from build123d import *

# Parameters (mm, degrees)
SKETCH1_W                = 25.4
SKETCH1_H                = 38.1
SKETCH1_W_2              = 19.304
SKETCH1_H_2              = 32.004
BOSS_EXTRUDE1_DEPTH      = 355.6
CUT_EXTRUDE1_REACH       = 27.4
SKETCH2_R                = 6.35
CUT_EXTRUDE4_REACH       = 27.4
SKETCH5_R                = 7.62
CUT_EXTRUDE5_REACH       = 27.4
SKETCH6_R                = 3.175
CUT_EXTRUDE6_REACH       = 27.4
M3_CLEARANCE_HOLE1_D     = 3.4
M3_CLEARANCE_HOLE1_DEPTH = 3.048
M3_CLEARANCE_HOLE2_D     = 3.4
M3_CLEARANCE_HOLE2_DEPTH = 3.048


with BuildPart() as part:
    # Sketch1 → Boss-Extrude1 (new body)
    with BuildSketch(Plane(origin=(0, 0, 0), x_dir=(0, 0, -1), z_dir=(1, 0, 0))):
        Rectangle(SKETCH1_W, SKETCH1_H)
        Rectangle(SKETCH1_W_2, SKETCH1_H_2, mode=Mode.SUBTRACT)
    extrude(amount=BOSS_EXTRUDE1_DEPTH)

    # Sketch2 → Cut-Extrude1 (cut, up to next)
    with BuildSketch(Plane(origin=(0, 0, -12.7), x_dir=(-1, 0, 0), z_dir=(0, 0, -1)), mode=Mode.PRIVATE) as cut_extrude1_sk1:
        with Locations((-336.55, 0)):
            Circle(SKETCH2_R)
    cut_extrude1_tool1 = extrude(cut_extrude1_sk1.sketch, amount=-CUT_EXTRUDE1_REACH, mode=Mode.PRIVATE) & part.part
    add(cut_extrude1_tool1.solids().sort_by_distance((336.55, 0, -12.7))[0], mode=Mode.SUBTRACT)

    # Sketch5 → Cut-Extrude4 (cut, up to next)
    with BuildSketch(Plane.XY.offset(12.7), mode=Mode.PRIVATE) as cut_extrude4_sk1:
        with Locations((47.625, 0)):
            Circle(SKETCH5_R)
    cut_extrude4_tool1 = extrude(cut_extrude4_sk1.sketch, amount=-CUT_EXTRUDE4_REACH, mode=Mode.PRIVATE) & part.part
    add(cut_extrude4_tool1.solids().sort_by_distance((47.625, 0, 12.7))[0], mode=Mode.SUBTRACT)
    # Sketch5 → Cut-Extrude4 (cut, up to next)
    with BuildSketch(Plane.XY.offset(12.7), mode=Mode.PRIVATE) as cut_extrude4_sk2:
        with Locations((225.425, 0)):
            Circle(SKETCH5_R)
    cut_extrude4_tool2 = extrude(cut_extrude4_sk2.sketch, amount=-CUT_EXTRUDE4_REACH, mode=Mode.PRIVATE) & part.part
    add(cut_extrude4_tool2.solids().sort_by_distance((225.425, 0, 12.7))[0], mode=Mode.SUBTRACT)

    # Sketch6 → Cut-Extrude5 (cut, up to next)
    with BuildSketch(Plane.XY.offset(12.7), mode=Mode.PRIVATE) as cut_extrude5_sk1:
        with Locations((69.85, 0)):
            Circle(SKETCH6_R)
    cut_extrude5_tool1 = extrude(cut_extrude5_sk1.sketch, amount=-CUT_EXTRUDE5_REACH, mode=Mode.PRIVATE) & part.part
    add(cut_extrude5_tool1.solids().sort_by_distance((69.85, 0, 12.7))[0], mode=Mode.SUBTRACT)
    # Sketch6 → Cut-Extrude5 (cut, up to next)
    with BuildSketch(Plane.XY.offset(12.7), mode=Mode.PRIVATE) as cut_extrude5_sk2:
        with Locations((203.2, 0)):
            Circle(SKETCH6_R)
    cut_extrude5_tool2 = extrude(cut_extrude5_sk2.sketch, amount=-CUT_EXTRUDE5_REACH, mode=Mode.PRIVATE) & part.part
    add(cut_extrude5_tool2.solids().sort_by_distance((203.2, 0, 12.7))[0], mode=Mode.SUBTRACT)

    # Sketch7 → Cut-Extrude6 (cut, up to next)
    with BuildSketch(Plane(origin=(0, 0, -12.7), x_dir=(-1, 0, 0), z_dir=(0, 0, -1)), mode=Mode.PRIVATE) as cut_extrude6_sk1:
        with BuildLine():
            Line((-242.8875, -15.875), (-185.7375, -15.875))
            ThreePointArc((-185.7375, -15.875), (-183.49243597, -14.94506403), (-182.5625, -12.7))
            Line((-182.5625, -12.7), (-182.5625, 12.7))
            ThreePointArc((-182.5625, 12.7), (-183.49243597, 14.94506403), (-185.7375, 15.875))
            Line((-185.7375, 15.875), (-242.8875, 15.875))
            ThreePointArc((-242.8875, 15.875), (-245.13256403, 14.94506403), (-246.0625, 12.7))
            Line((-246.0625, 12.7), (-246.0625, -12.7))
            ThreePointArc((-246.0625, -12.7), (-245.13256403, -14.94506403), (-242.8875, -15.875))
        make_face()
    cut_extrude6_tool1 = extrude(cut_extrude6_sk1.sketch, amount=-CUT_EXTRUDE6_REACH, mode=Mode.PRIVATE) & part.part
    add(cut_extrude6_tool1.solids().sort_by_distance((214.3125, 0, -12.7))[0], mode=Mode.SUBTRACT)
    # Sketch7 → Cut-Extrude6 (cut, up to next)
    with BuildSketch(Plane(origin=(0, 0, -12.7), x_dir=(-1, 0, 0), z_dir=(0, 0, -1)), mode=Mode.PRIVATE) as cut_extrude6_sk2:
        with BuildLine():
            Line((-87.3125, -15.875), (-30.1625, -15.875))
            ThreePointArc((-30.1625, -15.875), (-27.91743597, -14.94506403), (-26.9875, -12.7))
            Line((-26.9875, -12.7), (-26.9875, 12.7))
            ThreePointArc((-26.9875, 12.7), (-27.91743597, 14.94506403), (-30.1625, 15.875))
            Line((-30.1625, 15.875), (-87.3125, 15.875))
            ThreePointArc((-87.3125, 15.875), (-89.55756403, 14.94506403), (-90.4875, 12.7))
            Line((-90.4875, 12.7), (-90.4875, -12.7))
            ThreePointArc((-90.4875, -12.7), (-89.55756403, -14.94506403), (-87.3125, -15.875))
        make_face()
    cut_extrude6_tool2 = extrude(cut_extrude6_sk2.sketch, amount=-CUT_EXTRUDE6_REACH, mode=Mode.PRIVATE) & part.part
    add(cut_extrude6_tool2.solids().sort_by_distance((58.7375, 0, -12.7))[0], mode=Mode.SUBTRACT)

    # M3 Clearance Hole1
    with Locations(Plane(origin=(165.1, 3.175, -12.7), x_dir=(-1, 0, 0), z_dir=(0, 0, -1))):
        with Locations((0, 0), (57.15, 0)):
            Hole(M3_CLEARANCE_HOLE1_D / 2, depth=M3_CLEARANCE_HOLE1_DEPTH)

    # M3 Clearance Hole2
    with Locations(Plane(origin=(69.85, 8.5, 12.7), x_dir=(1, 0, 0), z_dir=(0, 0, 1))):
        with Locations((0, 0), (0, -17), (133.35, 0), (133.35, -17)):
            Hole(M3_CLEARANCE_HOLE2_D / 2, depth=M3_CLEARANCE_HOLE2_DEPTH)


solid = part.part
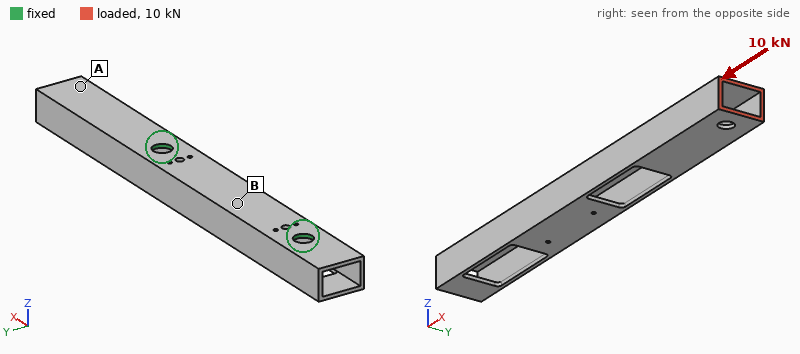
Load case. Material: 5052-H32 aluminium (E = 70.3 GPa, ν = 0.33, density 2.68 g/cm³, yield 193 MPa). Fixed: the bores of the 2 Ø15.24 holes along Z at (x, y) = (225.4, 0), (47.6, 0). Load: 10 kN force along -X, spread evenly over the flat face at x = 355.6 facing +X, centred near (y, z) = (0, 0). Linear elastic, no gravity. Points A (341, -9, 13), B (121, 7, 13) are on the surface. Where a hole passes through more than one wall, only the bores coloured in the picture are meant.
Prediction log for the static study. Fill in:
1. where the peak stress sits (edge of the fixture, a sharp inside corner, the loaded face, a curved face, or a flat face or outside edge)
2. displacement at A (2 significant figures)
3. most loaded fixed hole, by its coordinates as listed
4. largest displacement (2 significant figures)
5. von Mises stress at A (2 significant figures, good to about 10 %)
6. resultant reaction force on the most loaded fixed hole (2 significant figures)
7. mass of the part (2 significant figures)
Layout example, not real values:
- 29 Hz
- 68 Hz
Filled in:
- a curved face
- 0.50 mm
- (225.4, 0)
- 0.59 mm
- 29 MPa
- 7.0 kN
- 300 g
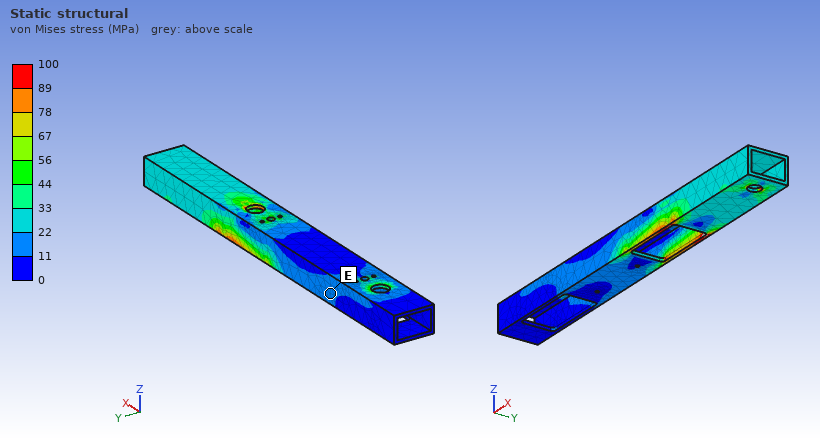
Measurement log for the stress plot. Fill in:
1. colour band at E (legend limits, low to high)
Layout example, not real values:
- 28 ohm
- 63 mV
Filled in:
- 11 to 22 MPa
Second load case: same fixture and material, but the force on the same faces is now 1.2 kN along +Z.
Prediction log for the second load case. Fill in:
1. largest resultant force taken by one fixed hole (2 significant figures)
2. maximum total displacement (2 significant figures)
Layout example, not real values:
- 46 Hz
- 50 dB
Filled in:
- 4.1 kN
- 1.3 mm
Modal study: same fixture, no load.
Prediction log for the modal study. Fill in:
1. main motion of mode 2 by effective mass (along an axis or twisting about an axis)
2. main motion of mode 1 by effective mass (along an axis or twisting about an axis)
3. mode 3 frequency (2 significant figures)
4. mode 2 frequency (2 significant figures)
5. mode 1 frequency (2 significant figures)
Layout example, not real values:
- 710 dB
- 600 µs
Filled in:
- along Y
- along Z
- 1500 Hz
- 1100 Hz
- 790 Hz
